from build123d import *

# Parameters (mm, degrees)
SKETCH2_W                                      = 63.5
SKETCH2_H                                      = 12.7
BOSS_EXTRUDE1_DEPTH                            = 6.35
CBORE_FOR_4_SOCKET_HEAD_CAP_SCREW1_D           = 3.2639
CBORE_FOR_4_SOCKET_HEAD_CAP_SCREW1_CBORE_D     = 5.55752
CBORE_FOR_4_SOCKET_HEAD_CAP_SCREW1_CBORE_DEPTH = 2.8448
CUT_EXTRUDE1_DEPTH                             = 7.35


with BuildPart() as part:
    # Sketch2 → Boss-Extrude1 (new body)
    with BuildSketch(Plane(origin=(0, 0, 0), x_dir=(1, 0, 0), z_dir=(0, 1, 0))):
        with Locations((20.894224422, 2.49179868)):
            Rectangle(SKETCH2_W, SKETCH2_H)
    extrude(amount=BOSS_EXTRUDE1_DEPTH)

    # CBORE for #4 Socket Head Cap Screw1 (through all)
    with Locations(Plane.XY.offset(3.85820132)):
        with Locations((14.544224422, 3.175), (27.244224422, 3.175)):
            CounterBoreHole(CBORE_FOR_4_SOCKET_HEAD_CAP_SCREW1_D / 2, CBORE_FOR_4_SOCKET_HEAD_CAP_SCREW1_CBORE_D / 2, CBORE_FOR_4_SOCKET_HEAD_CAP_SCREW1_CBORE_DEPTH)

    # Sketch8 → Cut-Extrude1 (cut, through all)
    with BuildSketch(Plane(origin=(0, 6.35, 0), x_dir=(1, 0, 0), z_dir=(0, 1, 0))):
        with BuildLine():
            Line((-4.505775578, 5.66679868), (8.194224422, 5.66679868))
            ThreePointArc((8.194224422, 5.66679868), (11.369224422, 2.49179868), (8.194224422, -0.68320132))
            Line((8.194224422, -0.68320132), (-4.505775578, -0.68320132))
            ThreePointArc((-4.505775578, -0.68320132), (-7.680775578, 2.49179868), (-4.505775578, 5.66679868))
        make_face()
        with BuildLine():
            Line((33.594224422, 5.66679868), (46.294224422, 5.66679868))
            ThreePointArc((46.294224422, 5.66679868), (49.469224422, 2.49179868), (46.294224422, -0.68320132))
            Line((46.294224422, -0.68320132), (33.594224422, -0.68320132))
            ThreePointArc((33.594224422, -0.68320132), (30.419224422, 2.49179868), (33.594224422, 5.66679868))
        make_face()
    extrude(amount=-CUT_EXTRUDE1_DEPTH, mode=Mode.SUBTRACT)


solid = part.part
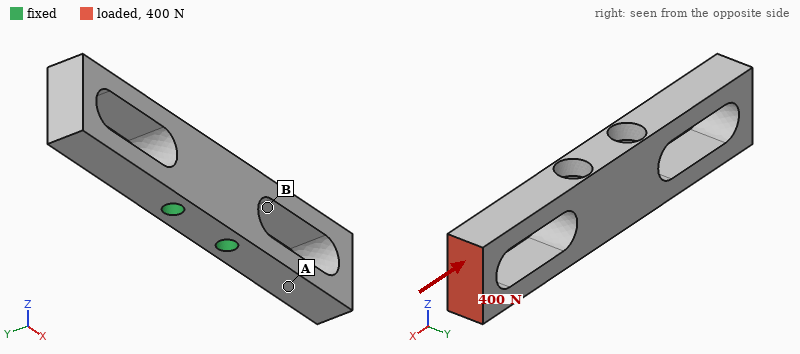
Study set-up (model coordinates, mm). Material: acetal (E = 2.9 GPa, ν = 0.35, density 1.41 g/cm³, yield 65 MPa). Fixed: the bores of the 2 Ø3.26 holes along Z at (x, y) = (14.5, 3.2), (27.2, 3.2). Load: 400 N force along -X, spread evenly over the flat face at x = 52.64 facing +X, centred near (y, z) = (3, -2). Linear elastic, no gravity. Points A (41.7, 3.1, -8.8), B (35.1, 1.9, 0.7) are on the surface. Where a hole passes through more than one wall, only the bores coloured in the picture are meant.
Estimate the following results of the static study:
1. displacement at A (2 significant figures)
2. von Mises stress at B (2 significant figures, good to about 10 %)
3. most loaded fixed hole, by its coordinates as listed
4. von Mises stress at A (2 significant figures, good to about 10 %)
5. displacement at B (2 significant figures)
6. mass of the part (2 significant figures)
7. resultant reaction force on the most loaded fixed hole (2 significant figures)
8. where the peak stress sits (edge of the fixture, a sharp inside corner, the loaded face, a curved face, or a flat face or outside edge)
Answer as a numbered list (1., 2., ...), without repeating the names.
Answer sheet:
1. 0.034 mm
2. 16 MPa
3. (27.2, 3.2)
4. 4.3 MPa
5. 0.095 mm
6. 4.8 g
7. 370 N
8. a curved face
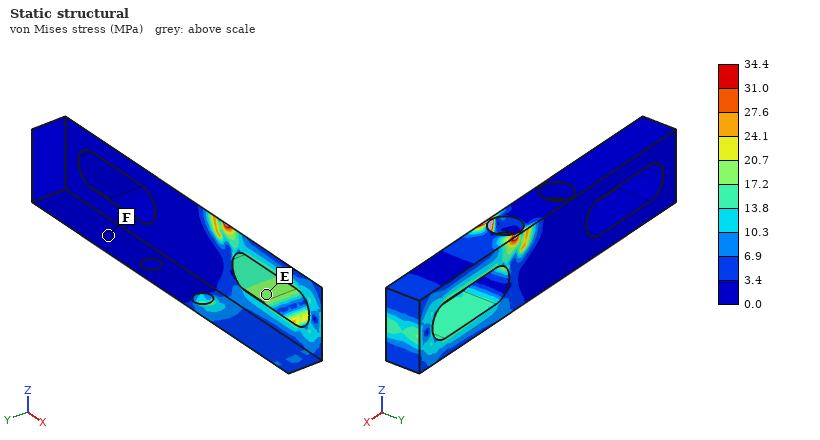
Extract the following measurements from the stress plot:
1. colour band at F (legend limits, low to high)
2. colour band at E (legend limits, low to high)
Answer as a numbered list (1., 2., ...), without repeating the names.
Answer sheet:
1. 0.0 to 3.4 MPa
2. 17.2 to 20.7 MPa
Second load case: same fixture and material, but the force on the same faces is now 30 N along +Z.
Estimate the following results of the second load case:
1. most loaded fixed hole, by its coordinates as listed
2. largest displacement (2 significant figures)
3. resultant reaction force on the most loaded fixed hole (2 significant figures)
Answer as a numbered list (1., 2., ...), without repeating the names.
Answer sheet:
1. (27.2, 3.2)
2. 0.30 mm
3. 41 N
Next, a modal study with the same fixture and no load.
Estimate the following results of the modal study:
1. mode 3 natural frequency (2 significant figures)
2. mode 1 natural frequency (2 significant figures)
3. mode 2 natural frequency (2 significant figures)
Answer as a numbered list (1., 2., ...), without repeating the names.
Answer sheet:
1. 1900 Hz
2. 1800 Hz
3. 1800 Hz
